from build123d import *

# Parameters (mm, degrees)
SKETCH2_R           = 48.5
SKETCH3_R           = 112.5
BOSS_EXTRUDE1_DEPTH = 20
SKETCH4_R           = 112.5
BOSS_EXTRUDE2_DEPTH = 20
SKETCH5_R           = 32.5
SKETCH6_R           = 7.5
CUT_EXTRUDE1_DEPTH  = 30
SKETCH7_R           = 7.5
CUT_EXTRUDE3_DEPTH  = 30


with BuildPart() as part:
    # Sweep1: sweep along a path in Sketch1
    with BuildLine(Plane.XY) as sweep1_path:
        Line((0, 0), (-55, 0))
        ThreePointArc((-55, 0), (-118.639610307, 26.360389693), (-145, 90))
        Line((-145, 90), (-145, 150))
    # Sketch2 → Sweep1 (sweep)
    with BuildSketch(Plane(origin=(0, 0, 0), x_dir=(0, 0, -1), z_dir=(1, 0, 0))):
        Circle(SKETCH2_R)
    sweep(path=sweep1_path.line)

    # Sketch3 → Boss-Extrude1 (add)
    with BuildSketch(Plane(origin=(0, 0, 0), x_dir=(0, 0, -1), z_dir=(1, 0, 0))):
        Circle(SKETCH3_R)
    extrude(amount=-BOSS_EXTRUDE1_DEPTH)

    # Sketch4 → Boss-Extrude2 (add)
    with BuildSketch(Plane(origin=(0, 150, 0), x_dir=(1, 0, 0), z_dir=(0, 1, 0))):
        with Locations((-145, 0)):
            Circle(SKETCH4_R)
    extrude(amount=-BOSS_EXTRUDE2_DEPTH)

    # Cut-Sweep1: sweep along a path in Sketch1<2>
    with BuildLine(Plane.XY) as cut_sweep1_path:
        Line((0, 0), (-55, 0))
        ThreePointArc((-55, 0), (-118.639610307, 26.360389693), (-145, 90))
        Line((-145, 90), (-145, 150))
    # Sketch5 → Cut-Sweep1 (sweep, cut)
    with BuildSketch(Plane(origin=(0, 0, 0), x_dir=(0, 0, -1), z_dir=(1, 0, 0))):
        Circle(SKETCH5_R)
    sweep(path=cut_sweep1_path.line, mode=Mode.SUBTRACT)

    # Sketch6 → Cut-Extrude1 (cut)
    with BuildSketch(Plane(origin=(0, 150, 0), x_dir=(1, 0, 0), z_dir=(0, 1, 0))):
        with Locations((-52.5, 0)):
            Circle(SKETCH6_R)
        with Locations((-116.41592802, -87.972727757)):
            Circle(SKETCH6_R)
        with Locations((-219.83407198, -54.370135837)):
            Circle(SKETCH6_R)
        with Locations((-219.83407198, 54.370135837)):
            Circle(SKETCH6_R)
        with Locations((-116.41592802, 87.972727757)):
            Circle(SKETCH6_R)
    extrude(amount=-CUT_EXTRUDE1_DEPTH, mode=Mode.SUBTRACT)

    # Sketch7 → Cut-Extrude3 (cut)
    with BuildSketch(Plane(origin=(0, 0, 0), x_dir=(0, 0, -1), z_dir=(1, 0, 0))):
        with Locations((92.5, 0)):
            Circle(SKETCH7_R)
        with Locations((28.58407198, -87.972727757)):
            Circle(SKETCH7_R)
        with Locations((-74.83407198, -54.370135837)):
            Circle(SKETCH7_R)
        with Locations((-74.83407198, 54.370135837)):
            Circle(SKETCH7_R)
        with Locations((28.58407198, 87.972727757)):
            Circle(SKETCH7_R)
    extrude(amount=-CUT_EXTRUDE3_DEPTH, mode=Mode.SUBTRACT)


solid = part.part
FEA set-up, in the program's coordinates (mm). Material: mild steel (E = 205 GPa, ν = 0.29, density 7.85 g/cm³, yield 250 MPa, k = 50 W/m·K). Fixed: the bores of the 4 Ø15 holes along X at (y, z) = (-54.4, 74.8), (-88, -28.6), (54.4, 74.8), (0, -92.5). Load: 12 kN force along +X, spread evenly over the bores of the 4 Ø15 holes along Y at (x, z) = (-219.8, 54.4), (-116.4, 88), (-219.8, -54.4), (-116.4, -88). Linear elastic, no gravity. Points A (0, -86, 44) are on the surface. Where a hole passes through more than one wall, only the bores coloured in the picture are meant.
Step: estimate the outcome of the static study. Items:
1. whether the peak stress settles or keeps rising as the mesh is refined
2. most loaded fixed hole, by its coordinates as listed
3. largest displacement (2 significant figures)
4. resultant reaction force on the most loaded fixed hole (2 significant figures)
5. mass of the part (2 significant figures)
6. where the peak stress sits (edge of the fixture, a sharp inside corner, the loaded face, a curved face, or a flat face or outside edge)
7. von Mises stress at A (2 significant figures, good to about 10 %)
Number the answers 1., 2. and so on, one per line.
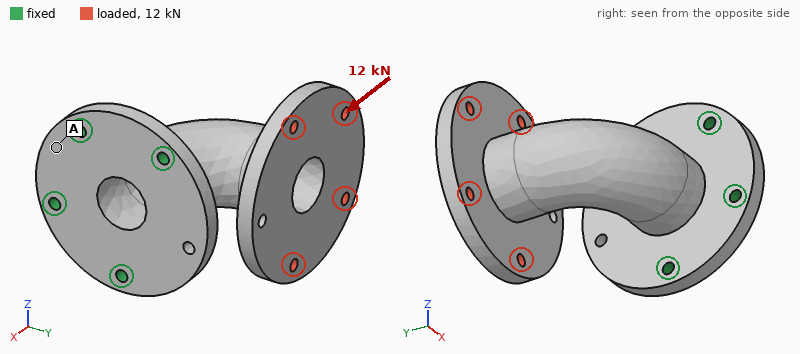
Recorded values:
1. keeps rising
2. (54.4, 74.8)
3. 0.27 mm
4. 15 kN
5. 18 kg
6. edge of the fixture
7. 8.4 MPa
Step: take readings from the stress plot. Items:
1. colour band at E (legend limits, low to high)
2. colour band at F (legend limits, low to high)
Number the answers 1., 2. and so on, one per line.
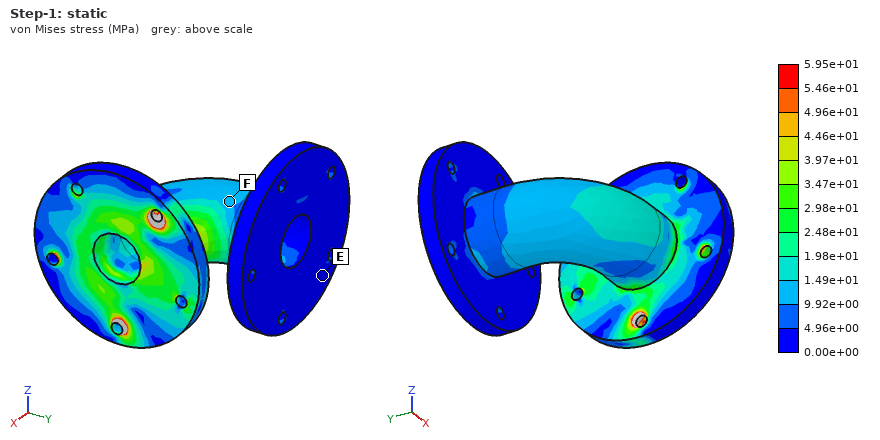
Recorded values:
1. 0.00e+00 to 4.96e+00 MPa
2. 9.92e+00 to 1.49e+01 MPa
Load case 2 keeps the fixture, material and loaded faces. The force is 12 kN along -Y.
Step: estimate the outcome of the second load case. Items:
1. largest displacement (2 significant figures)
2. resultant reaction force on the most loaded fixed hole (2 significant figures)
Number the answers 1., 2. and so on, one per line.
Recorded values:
1. 0.25 mm
2. 12 kN
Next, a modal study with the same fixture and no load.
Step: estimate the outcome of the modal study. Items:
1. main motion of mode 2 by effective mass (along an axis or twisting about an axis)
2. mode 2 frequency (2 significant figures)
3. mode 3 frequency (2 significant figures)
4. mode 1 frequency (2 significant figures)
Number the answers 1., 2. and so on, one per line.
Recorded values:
1. along Z
2. 520 Hz
3. 1100 Hz
4. 400 Hz
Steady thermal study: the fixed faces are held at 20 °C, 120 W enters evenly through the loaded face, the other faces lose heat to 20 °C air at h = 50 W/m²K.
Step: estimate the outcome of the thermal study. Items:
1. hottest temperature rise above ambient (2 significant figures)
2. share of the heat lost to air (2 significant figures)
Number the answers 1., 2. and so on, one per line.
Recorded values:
1. 33 K
2. 97 %
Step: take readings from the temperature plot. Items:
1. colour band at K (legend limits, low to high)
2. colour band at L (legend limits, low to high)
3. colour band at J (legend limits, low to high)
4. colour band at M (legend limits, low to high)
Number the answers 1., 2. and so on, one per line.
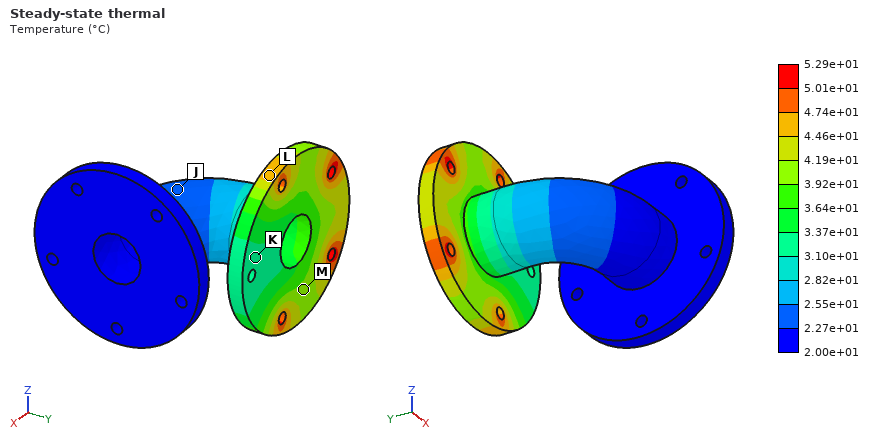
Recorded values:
1. 3.10e+01 to 3.37e+01 °C
2. 4.46e+01 to 4.74e+01 °C
3. 2.27e+01 to 2.55e+01 °C
4. 3.92e+01 to 4.19e+01 °C
